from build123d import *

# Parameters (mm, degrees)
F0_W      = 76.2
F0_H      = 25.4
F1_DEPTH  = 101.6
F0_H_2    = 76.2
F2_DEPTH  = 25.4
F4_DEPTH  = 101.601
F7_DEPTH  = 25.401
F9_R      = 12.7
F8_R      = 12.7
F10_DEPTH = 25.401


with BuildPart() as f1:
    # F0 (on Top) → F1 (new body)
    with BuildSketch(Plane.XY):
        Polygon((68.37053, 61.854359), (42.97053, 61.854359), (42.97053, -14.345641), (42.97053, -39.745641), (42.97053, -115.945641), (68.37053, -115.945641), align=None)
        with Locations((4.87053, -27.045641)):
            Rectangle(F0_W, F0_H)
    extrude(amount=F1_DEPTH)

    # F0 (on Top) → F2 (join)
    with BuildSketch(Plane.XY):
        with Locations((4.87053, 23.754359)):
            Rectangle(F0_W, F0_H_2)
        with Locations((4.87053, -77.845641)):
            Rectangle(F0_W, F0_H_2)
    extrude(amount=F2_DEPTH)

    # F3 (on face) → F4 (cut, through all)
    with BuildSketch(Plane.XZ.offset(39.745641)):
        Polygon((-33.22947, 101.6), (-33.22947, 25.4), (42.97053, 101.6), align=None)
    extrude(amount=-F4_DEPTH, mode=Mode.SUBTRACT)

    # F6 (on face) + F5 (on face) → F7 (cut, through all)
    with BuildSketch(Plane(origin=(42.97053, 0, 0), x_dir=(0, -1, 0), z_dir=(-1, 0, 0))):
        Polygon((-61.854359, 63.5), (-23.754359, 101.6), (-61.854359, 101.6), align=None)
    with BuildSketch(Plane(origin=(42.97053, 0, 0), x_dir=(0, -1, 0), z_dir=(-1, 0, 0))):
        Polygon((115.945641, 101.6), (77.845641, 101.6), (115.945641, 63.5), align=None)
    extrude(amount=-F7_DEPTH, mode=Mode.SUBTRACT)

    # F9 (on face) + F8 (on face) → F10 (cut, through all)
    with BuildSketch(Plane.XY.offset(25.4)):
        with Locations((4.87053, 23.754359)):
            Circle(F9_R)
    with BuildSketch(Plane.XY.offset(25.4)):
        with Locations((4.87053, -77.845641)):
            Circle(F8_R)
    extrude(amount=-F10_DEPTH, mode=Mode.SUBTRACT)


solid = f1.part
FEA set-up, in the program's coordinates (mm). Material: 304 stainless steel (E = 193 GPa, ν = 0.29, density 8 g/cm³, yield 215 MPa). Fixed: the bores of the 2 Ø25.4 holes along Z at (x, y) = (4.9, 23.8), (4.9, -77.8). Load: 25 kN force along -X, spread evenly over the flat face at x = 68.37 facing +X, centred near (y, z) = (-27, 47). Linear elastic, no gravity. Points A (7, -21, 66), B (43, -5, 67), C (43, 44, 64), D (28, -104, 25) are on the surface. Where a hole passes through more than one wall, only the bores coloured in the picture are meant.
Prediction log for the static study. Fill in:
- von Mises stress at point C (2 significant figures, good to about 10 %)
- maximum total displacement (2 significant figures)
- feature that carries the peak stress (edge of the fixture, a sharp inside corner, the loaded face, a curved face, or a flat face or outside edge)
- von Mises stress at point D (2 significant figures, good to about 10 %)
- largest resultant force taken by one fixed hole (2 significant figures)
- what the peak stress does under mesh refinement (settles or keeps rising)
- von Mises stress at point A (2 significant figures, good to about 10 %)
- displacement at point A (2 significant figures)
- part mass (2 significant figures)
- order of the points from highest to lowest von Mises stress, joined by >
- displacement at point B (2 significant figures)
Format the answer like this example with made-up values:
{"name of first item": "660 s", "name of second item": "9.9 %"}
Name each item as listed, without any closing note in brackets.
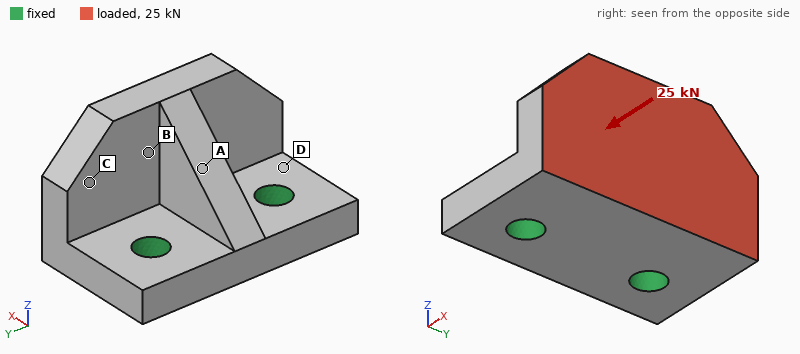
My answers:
{"von Mises stress at point C": "5.4 MPa", "maximum total displacement": "47 µm", "feature that carries the peak stress": "edge of the fixture", "von Mises stress at point D": "25 MPa", "largest resultant force taken by one fixed hole": "13 kN", "what the peak stress does under mesh refinement": "keeps rising", "von Mises stress at point A": "17 MPa", "displacement at point A": "21 µm", "part mass": "6.5 kg", "order of the points from highest to lowest von Mises stress, joined by >": "D > A > B > C", "displacement at point B": "26 µm"}
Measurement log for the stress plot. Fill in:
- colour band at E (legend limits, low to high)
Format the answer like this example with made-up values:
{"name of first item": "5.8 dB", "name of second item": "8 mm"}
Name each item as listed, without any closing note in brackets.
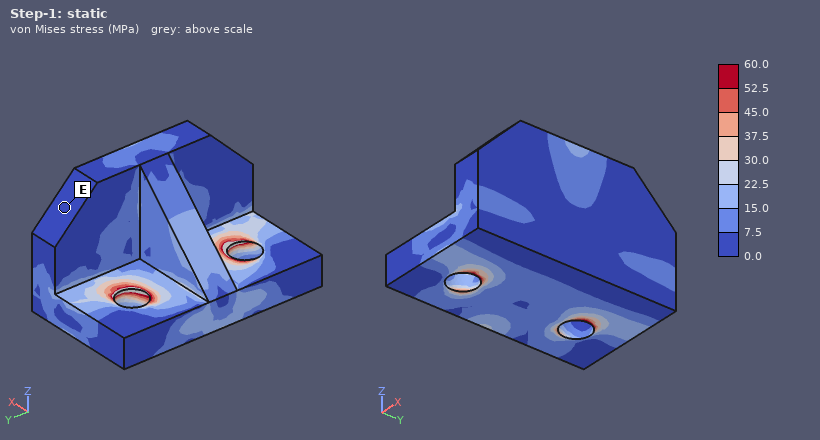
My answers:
{"colour band at E": "0.0 to 7.5 MPa"}
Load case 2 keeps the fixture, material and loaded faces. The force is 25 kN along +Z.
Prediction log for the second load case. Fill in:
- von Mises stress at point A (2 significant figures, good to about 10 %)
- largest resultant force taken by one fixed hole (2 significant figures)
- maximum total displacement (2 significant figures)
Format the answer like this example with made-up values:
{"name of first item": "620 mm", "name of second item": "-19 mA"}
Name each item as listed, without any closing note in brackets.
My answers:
{"von Mises stress at point A": "14 MPa", "largest resultant force taken by one fixed hole": "13 kN", "maximum total displacement": "61 µm"}
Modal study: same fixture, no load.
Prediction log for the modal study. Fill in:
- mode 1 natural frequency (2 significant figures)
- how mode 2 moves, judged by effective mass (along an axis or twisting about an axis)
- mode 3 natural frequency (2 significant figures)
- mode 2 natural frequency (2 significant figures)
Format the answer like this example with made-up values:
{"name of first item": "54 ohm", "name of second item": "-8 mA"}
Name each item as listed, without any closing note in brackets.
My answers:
{"mode 1 natural frequency": "2000 Hz", "how mode 2 moves, judged by effective mass": "along Y", "mode 3 natural frequency": "4500 Hz", "mode 2 natural frequency": "3100 Hz"}
